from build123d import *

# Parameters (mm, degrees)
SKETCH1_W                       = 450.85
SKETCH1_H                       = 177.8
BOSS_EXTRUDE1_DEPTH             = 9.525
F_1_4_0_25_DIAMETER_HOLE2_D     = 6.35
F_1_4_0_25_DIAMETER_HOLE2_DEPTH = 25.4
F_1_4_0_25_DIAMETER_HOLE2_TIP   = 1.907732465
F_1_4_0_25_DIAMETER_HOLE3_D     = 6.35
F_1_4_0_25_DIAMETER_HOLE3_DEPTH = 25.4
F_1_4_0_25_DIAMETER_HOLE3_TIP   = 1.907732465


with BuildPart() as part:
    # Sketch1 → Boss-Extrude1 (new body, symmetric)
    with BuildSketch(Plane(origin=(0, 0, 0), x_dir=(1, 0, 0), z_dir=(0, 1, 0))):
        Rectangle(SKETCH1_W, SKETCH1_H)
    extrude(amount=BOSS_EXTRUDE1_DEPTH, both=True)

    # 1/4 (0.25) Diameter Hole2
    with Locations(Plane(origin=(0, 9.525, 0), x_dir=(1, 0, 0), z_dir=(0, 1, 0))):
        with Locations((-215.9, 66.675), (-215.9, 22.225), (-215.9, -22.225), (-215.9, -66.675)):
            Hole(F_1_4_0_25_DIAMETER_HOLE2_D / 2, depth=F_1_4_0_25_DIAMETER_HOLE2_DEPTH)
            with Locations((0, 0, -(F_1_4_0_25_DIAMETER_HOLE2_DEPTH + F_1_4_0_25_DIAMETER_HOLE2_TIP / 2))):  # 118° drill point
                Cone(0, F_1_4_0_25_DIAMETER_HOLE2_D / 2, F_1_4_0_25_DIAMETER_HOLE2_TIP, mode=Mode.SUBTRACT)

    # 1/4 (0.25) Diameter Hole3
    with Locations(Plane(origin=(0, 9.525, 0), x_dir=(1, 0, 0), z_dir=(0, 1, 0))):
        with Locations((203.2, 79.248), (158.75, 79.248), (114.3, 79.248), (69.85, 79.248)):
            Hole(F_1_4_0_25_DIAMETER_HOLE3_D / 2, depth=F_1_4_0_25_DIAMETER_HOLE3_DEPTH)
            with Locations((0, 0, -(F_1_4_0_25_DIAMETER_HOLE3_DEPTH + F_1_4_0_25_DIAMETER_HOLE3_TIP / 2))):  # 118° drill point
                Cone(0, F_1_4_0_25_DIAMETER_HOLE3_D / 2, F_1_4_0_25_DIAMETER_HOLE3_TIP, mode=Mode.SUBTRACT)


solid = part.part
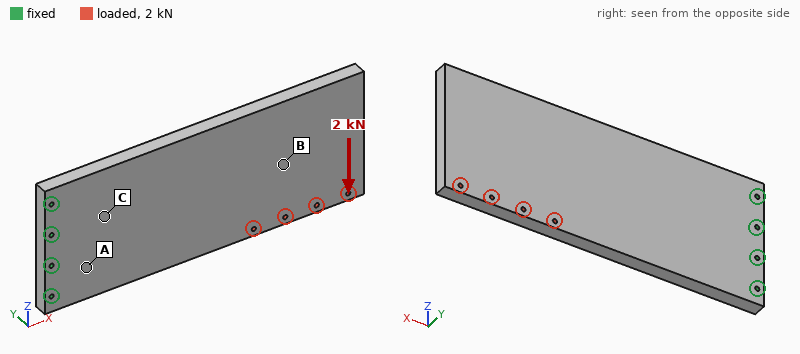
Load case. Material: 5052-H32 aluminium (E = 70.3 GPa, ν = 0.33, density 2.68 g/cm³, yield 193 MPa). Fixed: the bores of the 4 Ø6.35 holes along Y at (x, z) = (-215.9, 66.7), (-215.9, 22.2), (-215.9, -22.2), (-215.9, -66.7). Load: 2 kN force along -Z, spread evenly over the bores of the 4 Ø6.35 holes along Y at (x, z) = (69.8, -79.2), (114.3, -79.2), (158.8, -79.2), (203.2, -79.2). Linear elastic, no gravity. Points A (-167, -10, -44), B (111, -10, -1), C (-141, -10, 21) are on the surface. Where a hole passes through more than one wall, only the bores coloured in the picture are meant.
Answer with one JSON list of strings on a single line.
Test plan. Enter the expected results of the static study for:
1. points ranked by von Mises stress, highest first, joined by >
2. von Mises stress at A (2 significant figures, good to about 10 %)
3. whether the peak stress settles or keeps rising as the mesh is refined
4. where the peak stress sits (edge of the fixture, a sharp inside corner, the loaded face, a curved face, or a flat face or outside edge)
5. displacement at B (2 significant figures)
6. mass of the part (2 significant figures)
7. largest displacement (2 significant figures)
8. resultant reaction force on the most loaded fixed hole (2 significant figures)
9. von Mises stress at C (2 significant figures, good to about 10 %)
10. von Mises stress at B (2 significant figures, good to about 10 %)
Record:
["A > C > B", "3.5 MPa", "keeps rising", "edge of the fixture", "58 µm", "4.1 kg", "88 µm", "4.8 kN", "2.1 MPa", "1.0 MPa"]
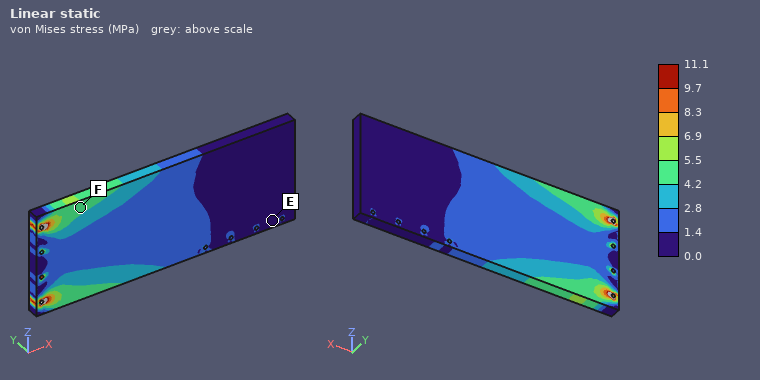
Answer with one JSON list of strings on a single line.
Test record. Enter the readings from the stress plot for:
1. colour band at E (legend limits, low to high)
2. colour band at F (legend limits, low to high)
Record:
["0.0 to 1.4 MPa", "4.2 to 5.5 MPa"]
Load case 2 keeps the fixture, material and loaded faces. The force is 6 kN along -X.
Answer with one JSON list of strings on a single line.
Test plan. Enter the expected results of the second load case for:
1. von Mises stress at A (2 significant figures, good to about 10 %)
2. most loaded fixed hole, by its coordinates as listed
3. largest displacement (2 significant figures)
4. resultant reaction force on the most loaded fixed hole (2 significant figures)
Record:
["4.3 MPa", "(-215.9, -66.7)", "87 µm", "4.7 kN"]
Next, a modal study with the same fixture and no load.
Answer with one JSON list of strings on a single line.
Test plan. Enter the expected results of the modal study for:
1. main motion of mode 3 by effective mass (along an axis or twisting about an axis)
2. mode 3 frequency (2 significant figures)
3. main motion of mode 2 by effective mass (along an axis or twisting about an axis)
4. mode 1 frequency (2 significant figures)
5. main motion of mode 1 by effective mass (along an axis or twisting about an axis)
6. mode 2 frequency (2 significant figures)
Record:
["along Y", "490 Hz", "twisting about X", "80 Hz", "along Y", "400 Hz"]
